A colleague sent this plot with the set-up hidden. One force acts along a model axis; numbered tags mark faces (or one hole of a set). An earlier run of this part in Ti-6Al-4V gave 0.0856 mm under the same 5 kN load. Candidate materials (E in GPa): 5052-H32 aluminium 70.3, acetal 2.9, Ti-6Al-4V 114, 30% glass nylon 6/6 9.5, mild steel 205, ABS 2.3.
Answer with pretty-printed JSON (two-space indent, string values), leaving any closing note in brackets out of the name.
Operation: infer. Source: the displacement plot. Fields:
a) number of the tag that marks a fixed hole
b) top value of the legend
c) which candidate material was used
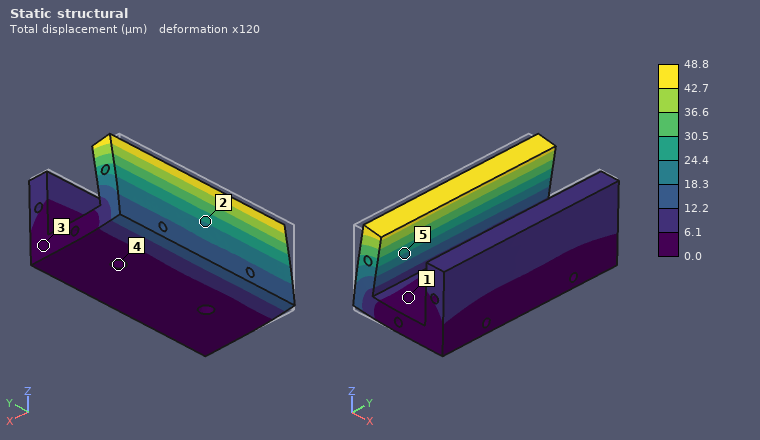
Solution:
{
  "number of the tag that marks a fixed hole": "4",
  "top value of the legend": "48.8 µm",
  "which candidate material was used": "mild steel"
}
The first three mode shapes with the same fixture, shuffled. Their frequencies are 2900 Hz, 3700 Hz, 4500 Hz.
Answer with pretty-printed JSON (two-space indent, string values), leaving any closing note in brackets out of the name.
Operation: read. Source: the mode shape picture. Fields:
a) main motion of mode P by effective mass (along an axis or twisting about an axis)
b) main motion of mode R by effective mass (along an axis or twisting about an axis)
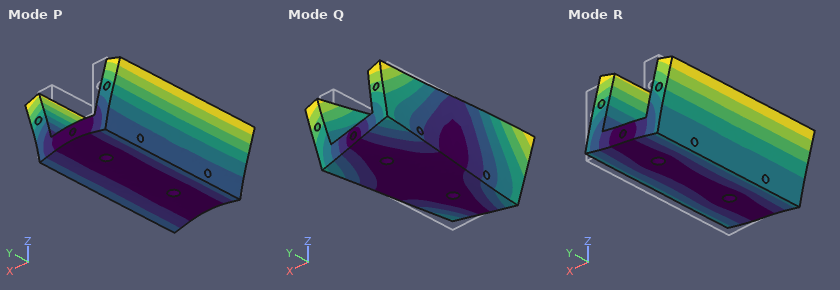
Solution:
{
  "main motion of mode P by effective mass": "along Z",
  "main motion of mode R by effective mass": "along X"
}
